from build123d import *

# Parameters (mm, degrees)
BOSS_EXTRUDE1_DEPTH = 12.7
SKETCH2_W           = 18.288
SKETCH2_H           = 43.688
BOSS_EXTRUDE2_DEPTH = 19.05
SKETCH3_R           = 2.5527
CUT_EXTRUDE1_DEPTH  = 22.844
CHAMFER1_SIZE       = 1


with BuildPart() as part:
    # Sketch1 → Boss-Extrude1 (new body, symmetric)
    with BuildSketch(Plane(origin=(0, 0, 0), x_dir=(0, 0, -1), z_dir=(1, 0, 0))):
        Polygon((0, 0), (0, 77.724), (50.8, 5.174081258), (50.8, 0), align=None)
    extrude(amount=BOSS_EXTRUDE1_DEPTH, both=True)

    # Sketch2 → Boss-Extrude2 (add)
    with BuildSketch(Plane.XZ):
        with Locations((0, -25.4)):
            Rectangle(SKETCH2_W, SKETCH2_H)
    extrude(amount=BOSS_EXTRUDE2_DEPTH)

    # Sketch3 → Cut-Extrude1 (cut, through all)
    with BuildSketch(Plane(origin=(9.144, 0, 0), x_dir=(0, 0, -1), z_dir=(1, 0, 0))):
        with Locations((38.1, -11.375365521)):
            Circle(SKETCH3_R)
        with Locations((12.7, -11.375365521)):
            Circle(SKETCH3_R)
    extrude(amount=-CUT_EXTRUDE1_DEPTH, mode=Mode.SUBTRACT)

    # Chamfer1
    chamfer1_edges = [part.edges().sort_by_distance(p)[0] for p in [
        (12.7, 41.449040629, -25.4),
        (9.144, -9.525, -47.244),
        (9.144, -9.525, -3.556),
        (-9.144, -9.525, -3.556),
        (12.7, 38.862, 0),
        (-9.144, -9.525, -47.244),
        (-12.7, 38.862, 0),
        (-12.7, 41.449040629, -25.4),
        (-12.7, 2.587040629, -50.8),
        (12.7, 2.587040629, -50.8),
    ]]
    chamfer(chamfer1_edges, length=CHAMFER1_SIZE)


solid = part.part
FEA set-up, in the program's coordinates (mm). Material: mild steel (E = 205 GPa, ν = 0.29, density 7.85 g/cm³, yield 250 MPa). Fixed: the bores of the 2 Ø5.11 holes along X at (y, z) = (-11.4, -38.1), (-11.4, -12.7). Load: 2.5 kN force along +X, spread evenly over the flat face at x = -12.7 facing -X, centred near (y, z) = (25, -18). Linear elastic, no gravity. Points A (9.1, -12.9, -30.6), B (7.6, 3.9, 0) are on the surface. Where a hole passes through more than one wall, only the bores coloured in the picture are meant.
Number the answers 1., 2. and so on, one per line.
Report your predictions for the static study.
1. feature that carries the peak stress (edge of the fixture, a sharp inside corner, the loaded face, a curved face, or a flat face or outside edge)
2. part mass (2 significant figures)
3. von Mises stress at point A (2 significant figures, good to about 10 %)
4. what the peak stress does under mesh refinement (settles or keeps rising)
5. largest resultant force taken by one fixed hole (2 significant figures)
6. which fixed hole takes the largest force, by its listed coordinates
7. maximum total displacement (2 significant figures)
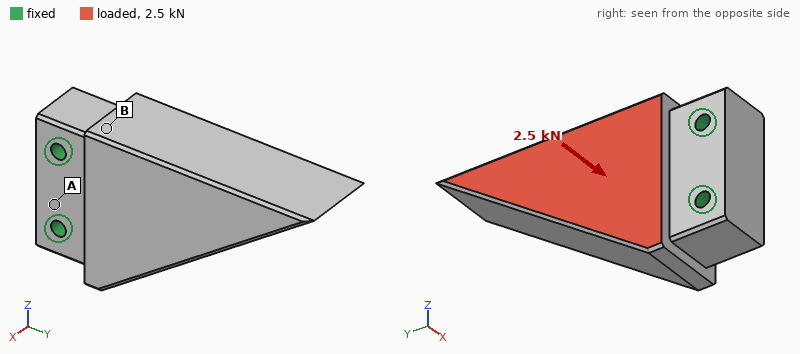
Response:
1. edge of the fixture
2. 530 g
3. 15 MPa
4. keeps rising
5. 1.7 kN
6. (-11.4, -12.7)
7. 33 µm
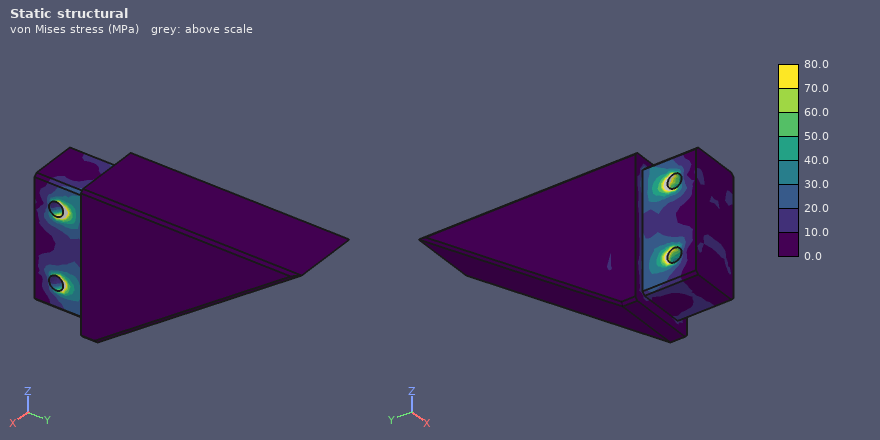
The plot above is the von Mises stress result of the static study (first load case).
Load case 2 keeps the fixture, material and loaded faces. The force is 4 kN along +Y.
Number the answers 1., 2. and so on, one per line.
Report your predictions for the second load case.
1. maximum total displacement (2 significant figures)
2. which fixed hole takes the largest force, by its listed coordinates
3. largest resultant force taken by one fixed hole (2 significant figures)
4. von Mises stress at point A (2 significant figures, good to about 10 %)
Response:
1. 23 µm
2. (-11.4, -12.7)
3. 3.0 kN
4. 6.3 MPa
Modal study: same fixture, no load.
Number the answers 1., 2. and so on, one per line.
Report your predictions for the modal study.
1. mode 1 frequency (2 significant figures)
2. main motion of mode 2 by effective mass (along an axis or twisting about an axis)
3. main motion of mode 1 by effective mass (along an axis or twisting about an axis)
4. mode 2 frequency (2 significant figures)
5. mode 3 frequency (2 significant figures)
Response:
1. 3000 Hz
2. along Z
3. along X
4. 5400 Hz
5. 11 kHz
